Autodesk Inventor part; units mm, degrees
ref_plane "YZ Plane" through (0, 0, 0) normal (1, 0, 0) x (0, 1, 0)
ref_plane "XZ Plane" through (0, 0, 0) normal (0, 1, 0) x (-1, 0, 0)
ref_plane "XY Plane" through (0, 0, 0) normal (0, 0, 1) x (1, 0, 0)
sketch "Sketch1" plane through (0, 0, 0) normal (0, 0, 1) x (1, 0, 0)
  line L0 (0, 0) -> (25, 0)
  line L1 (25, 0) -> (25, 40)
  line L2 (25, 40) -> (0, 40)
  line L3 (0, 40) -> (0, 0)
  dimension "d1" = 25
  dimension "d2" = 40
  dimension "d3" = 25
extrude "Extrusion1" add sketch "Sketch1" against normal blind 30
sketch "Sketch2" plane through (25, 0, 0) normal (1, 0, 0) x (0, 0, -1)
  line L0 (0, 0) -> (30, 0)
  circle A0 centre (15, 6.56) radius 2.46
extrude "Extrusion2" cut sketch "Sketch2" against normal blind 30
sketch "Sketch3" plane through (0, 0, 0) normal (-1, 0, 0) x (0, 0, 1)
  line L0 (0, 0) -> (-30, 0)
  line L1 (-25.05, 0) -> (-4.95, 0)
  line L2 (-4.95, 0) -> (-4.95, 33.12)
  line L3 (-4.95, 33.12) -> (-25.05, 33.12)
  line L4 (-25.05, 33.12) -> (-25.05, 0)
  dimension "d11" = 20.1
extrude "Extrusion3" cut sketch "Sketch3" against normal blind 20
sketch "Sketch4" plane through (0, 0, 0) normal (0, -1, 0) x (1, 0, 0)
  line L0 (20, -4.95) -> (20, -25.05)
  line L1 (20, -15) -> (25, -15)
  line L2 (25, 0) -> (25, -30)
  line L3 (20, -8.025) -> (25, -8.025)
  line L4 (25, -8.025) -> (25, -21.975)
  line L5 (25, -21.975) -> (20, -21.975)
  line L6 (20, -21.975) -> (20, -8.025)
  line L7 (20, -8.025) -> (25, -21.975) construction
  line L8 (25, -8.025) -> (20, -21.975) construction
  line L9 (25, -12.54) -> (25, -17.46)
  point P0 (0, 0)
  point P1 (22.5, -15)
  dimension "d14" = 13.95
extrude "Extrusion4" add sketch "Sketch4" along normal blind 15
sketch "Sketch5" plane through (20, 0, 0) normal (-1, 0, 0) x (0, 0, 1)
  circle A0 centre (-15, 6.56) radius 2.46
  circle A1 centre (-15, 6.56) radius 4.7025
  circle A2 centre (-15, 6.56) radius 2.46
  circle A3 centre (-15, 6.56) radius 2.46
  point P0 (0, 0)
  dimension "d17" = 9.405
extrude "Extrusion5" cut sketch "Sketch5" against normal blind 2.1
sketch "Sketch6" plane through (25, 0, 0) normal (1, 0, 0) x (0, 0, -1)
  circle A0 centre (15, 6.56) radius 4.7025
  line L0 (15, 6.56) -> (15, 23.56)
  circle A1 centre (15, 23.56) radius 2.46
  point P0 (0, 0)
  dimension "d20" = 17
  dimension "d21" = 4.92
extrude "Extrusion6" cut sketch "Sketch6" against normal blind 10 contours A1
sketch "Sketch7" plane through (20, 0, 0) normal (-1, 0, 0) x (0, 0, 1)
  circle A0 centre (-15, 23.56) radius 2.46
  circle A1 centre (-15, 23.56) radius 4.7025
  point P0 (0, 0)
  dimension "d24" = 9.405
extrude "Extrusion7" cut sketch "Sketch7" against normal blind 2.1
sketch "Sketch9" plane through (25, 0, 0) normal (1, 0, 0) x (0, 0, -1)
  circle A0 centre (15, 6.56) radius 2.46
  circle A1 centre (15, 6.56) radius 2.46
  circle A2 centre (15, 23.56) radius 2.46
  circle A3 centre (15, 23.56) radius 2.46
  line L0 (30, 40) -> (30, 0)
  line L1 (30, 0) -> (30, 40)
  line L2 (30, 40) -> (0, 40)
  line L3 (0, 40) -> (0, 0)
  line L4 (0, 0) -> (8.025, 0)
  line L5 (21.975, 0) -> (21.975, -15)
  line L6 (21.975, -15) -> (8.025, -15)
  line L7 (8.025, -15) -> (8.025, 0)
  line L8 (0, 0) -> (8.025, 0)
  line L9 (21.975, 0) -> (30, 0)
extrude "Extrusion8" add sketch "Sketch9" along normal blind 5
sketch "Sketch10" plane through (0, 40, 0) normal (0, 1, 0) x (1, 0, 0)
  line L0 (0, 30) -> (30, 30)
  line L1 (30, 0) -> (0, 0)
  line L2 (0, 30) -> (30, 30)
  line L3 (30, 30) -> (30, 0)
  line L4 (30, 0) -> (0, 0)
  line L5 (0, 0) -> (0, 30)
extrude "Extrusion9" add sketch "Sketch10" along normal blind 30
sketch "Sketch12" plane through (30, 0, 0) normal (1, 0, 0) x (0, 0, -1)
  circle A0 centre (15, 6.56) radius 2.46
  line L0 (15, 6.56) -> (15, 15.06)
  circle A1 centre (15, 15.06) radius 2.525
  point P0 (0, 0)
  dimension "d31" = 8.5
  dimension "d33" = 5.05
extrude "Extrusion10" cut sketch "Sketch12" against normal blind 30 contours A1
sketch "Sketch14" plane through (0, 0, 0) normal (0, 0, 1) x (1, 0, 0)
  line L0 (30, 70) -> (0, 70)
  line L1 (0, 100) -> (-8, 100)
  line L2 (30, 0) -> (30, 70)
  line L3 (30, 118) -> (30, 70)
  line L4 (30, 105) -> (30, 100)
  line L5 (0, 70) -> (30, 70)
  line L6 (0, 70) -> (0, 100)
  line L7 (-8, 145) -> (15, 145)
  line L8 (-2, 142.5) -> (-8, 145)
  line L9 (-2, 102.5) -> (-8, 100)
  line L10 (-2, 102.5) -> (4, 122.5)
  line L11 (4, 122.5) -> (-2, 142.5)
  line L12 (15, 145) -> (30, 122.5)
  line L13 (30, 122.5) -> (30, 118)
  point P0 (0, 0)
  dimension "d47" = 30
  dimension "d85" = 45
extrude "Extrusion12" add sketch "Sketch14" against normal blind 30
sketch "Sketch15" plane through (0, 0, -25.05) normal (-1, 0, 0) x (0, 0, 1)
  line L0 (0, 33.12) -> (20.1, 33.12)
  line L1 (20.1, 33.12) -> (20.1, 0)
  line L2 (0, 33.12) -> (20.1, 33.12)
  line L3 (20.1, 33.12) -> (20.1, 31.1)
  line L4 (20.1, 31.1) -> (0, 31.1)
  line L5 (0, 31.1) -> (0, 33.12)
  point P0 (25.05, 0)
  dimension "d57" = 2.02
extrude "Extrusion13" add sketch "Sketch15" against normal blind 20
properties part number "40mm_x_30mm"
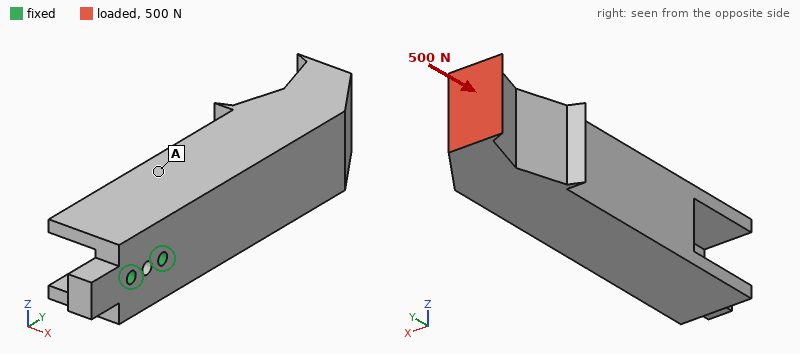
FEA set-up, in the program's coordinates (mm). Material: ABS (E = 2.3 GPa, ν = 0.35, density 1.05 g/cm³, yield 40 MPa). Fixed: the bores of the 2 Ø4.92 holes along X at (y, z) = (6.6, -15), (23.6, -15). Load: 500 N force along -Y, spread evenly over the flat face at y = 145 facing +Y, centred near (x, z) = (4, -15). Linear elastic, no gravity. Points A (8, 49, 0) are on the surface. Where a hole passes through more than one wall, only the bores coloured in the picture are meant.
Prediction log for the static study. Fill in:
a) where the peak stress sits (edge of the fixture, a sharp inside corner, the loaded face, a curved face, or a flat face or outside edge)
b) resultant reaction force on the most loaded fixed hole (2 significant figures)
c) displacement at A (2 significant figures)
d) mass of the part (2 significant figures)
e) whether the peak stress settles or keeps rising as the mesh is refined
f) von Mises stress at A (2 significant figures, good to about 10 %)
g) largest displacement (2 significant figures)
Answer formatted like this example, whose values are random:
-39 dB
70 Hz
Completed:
edge of the fixture
520 N
0.24 mm
120 g
keeps rising
1.4 MPa
1.3 mm
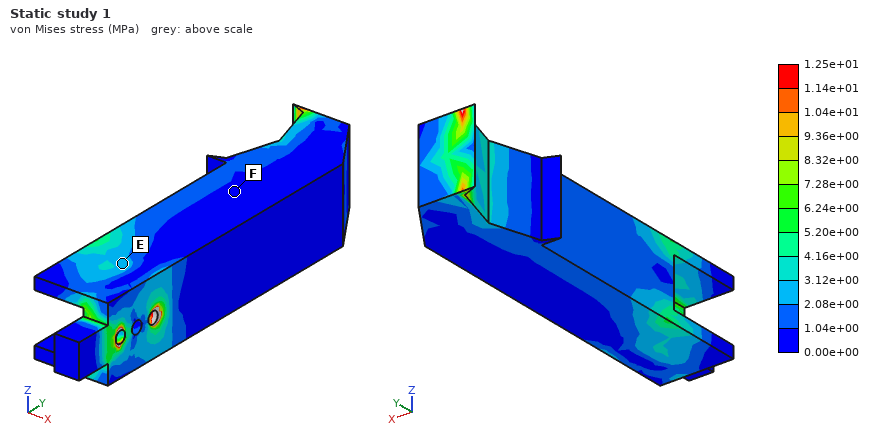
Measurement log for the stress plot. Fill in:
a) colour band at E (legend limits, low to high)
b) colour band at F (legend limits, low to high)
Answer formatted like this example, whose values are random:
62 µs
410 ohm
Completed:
2.08e+00 to 3.12e+00 MPa
0.00e+00 to 1.04e+00 MPa
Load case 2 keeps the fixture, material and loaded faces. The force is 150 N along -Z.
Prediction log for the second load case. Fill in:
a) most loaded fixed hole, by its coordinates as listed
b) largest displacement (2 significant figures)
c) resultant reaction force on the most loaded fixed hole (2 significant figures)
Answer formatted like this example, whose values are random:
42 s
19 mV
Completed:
(23.6, -15)
1.6 mm
940 N
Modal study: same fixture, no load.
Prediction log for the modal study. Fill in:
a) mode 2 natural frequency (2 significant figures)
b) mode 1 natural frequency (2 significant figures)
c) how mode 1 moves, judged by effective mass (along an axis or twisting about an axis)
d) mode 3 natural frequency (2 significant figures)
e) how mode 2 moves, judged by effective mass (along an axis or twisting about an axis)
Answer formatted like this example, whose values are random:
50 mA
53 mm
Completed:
290 Hz
250 Hz
along X
880 Hz
along Z
